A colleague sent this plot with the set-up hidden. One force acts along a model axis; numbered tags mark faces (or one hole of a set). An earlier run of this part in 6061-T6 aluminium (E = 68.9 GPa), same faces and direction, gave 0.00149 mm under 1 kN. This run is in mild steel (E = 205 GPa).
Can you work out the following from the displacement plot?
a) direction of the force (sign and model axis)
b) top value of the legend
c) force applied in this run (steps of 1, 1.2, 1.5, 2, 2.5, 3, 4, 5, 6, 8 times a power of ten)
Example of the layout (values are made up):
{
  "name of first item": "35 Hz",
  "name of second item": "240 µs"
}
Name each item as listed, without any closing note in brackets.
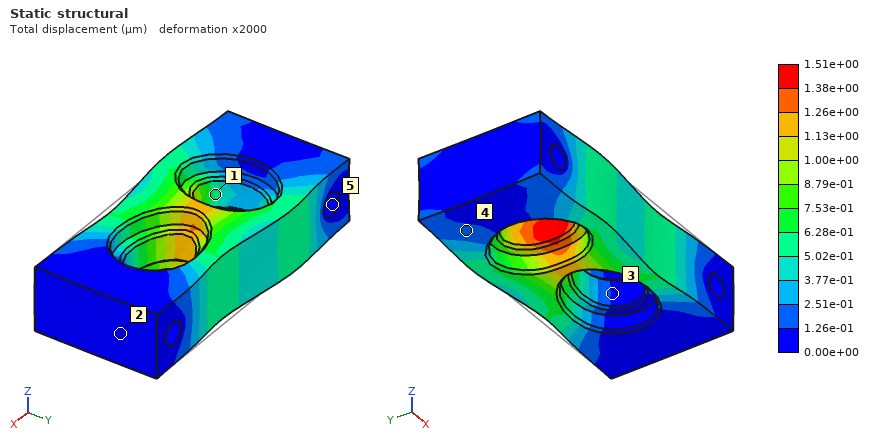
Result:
{
  "direction of the force": "-X",
  "top value of the legend": "1.51e+00 µm",
  "force applied in this run": "3 kN"
}
